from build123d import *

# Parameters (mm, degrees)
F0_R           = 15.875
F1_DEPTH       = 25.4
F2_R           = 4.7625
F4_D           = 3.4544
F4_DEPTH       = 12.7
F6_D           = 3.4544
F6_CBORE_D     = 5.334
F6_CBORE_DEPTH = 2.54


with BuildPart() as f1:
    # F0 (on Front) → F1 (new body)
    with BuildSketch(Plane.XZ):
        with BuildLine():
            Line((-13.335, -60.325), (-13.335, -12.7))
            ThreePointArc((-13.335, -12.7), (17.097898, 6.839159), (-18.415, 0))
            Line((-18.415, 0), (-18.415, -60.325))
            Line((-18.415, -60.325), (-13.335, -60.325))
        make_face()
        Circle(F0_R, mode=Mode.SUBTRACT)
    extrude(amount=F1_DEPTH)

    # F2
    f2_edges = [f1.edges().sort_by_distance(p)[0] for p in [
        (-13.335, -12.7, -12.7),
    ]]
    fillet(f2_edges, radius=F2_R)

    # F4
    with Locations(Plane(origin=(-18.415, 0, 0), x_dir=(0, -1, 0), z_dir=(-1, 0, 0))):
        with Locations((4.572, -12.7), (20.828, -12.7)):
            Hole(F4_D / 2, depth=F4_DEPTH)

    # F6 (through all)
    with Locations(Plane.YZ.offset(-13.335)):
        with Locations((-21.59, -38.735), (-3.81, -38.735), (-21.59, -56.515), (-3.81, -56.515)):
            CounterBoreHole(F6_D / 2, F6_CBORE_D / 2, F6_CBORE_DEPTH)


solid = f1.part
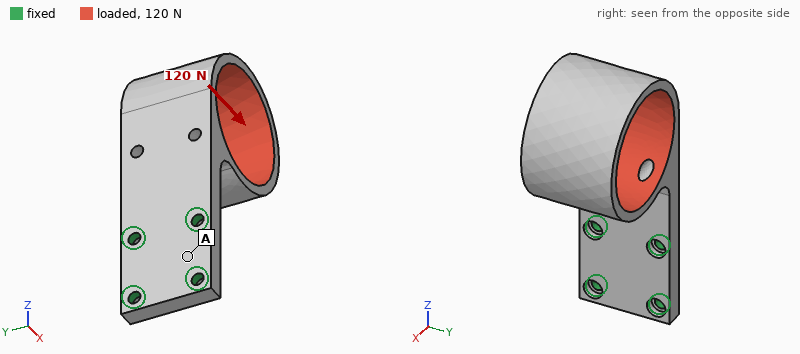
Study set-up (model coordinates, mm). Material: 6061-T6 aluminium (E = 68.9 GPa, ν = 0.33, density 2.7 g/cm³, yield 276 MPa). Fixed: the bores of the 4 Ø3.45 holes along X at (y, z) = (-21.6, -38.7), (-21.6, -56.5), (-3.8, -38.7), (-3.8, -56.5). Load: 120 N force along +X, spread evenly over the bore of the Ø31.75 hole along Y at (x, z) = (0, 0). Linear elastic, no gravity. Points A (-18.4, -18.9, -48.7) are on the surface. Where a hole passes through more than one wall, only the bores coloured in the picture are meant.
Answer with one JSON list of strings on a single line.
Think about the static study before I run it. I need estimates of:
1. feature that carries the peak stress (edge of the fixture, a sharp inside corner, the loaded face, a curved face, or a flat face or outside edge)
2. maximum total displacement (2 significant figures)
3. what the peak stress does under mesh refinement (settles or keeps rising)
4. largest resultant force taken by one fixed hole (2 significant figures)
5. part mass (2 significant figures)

["edge of the fixture", "0.29 mm", "keeps rising", "220 N", "36 g"]
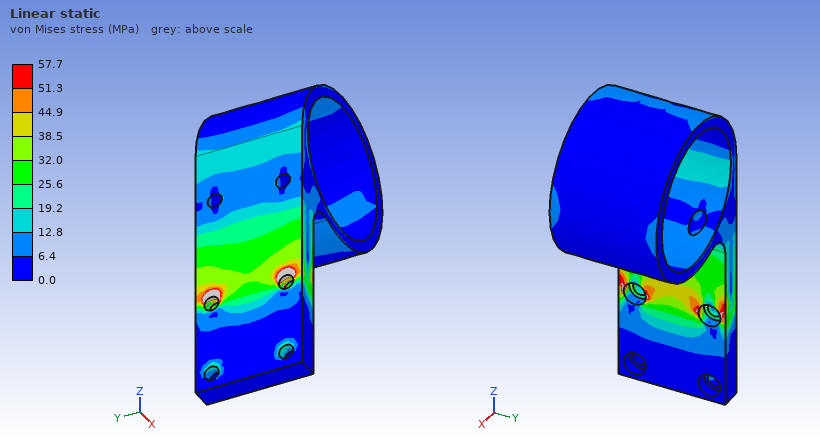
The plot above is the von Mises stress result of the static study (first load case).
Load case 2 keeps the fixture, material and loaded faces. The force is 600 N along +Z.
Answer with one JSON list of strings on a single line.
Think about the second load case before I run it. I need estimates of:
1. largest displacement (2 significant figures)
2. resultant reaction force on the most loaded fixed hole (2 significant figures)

["0.91 mm", "430 N"]
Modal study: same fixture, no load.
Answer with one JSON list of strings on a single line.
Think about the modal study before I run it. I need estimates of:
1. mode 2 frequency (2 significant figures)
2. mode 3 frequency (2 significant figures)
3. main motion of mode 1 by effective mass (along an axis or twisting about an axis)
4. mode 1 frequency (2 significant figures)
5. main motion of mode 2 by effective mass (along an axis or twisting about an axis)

["1900 Hz", "3000 Hz", "along X", "750 Hz", "along Y"]
